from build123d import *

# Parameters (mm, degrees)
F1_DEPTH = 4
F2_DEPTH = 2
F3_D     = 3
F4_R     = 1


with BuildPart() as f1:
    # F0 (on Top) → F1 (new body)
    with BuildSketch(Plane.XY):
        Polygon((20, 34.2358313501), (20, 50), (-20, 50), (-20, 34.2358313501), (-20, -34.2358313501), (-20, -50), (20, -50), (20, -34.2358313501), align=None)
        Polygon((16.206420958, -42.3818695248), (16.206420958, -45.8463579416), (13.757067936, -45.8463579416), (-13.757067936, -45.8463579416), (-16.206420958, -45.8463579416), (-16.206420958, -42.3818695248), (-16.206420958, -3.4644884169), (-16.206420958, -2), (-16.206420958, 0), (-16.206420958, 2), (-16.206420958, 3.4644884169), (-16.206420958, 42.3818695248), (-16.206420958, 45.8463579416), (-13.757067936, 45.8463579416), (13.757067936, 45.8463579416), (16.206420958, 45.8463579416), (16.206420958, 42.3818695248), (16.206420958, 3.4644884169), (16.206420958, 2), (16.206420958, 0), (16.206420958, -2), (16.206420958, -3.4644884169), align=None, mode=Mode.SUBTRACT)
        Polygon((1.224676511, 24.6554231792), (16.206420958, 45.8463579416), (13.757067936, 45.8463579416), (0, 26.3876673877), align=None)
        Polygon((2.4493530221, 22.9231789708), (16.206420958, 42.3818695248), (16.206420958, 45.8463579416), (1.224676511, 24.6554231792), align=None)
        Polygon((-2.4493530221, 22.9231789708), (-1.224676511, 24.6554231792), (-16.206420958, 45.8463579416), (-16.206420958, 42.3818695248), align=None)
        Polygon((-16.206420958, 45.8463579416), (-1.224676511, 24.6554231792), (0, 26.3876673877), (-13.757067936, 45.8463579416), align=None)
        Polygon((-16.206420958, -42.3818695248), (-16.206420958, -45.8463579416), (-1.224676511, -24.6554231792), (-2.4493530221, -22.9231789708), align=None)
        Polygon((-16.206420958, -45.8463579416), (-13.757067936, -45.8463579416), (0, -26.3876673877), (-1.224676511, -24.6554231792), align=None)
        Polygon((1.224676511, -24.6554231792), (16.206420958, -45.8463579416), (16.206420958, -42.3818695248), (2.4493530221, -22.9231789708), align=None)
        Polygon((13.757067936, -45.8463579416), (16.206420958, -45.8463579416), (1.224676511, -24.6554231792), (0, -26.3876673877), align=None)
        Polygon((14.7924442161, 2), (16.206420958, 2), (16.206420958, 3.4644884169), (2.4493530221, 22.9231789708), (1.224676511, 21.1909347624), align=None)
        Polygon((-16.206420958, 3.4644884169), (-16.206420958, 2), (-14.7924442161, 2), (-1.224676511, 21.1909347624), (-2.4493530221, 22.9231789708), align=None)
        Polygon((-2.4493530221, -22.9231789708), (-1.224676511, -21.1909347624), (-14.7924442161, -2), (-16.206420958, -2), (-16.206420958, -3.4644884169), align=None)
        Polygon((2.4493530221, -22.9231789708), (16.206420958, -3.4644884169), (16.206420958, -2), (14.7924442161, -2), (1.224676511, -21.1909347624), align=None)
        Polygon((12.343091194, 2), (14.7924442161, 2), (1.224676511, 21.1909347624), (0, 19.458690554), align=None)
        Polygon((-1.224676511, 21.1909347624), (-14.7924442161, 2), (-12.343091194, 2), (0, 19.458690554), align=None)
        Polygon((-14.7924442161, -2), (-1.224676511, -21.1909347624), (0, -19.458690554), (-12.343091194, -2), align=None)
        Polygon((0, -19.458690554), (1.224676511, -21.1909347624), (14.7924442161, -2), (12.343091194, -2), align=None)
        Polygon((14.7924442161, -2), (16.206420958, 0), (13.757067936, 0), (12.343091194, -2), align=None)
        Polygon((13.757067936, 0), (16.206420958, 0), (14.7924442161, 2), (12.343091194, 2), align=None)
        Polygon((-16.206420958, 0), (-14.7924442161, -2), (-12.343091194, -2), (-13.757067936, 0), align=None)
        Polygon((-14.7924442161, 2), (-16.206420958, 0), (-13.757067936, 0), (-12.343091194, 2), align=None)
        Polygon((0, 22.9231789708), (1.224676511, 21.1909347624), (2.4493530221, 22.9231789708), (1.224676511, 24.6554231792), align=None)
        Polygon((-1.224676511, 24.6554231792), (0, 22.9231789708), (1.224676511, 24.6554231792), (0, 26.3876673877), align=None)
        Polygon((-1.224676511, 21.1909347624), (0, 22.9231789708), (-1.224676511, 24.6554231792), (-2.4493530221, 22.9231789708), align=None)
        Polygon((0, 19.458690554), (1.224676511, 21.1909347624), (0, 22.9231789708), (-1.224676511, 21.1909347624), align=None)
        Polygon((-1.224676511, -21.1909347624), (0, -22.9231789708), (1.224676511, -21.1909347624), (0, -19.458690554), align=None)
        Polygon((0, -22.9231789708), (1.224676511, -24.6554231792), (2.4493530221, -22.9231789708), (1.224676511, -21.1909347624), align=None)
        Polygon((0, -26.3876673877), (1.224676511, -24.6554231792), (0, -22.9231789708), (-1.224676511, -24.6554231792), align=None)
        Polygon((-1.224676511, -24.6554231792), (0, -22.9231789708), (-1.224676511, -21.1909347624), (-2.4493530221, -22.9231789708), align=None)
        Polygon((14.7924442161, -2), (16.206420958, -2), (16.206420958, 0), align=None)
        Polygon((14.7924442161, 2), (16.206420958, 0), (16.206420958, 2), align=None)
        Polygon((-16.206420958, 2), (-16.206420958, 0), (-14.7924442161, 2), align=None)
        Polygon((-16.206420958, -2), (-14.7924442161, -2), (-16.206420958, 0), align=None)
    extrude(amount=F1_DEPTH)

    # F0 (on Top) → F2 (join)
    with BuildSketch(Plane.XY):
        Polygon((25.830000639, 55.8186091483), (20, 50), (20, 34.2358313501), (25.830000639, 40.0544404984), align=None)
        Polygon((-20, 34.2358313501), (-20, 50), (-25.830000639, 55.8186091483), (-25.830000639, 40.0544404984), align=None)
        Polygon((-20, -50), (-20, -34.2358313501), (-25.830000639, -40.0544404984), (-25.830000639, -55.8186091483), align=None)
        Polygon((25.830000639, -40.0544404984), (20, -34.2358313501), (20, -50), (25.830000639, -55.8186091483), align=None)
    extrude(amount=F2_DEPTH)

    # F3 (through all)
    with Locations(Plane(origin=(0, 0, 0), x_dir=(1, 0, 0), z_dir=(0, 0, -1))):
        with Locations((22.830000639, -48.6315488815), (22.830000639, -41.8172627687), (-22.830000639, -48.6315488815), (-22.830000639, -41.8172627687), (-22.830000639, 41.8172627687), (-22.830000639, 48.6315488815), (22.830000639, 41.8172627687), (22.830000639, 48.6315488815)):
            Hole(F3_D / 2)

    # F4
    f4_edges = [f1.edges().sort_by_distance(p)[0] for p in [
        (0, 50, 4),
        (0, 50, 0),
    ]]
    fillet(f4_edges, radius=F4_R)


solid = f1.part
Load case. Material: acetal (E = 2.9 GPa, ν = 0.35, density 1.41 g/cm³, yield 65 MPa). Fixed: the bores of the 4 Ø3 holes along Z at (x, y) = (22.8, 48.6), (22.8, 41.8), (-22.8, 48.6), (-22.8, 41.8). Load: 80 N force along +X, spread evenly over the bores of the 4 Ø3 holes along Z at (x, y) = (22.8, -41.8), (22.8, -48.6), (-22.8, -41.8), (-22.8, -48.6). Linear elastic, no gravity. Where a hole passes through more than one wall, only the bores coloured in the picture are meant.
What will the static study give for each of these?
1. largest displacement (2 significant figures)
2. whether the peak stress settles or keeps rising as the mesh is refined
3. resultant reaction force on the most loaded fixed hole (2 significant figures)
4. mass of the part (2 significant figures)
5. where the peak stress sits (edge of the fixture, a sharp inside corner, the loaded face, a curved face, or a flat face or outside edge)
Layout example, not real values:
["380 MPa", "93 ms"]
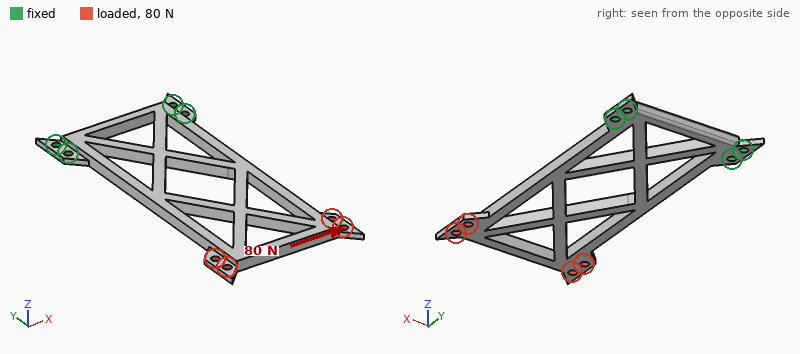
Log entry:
["1.4 mm", "keeps rising", "130 N", "11 g", "edge of the fixture"]
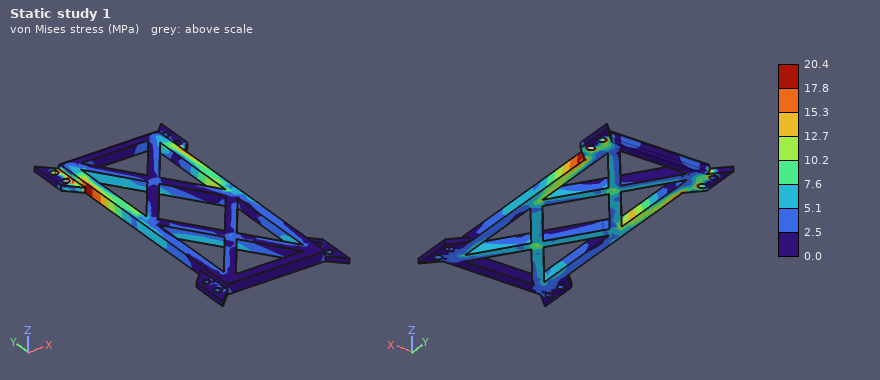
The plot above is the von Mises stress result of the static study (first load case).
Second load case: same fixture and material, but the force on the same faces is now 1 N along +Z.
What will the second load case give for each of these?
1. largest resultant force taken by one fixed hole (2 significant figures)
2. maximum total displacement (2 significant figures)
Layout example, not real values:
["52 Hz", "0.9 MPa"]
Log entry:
["5.0 N", "1.4 mm"]
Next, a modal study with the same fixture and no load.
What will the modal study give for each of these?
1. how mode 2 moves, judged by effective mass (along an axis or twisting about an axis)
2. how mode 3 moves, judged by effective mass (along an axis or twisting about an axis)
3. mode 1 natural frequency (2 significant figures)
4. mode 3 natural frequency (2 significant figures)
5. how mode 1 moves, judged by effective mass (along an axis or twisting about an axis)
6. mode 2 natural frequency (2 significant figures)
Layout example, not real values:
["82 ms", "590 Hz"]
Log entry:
["twisting about Y", "along Z", "78 Hz", "510 Hz", "along Z", "290 Hz"]
